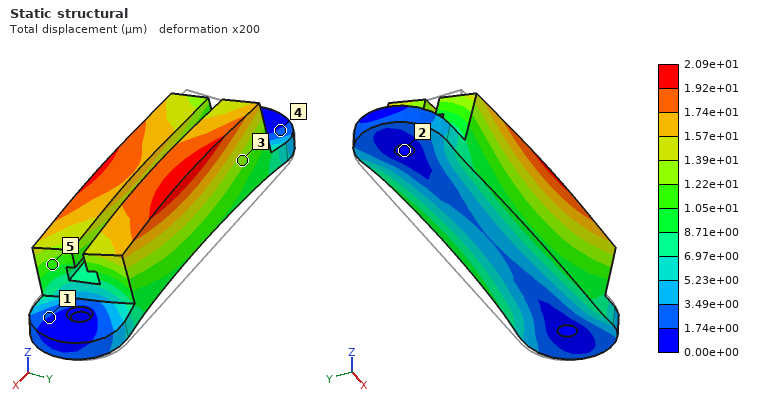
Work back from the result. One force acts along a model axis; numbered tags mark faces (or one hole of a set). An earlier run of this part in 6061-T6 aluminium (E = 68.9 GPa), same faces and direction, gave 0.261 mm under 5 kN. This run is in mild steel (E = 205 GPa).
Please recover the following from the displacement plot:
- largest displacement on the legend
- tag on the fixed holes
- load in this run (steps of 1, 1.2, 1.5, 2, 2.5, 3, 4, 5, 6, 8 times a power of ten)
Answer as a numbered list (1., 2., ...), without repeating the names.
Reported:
1. 2.09e+01 µm
2. 2
3. 1.2 kN
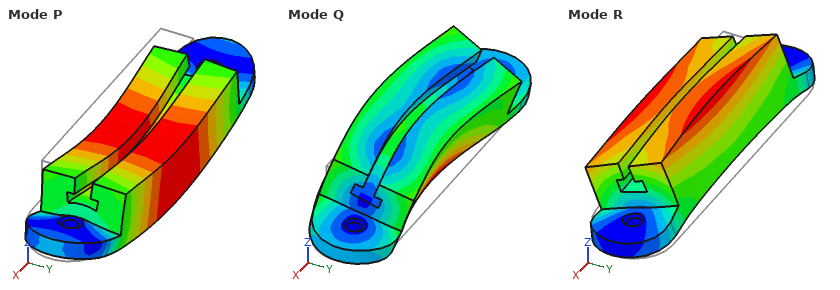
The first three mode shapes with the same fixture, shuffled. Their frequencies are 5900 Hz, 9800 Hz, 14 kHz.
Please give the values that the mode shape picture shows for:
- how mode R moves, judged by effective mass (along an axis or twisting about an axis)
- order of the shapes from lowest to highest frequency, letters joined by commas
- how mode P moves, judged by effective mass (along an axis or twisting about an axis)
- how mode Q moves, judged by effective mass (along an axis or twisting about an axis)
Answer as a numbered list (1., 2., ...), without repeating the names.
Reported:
1. along Y
2. R, P, Q
3. along Z
4. along Y
